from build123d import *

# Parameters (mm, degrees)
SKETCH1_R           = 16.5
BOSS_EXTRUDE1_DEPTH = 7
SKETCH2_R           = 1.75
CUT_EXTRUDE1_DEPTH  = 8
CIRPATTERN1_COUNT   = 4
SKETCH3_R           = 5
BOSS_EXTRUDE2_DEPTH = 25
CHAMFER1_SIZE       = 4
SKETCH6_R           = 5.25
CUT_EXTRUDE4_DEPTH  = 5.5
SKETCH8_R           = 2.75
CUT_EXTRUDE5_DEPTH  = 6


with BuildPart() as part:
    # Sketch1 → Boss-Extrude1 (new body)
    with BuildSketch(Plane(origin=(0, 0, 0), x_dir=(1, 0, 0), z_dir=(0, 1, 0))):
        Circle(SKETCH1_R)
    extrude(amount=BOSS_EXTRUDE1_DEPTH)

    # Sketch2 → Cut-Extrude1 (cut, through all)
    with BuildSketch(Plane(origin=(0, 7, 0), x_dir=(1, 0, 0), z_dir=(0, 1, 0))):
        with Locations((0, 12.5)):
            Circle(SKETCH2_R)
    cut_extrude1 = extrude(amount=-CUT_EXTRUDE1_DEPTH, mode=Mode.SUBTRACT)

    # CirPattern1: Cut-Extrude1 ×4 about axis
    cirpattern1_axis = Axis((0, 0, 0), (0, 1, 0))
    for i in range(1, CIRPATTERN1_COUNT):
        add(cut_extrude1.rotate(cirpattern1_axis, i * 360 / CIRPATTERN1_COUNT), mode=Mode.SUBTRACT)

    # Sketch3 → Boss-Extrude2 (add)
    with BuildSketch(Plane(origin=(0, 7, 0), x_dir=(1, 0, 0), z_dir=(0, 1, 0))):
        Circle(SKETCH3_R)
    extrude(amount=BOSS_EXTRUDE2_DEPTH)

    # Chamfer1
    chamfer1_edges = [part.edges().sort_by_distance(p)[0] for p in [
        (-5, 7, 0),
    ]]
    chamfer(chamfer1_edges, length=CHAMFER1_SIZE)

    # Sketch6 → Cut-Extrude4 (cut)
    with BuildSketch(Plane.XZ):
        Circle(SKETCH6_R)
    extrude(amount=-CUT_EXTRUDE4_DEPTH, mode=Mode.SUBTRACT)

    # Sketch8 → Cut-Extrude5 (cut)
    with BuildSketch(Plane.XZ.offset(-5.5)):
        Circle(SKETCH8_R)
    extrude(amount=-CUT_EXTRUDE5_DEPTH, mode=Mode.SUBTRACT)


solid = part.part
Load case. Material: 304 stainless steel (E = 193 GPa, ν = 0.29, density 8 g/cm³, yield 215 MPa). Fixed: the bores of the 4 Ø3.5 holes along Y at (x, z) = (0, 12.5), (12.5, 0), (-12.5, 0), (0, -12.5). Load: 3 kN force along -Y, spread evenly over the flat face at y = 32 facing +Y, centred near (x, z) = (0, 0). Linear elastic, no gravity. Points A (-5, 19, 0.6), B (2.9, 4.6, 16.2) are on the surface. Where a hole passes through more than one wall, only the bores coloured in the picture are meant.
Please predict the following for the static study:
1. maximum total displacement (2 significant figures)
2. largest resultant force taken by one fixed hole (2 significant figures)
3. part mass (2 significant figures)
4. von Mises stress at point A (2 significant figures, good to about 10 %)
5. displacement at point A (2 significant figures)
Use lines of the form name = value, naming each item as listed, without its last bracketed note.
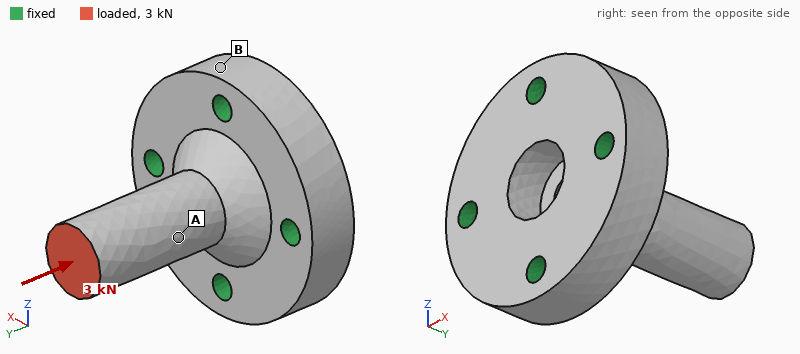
maximum total displacement = 6.4 µm
largest resultant force taken by one fixed hole = 840 N
part mass = 59 g
von Mises stress at point A = 38 MPa
displacement at point A = 3.8 µm
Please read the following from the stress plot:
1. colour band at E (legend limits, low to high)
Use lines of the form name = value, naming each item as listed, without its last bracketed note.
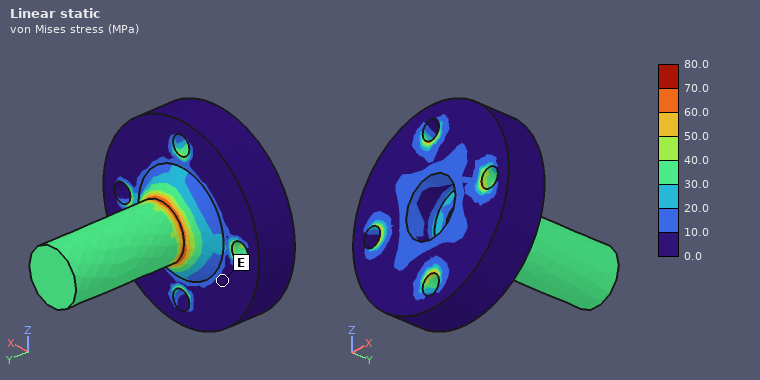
colour band at E = 0.0 to 10.0 MPa
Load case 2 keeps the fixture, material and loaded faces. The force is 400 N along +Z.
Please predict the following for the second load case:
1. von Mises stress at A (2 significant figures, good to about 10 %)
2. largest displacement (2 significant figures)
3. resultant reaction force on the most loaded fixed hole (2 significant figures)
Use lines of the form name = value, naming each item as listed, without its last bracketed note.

von Mises stress at A = 12 MPa
largest displacement = 24 µm
resultant reaction force on the most loaded fixed hole = 530 N
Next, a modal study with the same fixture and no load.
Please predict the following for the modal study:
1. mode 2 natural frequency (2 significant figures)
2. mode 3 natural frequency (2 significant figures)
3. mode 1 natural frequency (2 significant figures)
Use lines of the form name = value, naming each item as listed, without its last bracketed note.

mode 2 natural frequency = 10 kHz
mode 3 natural frequency = 32 kHz
mode 1 natural frequency = 10 kHz
